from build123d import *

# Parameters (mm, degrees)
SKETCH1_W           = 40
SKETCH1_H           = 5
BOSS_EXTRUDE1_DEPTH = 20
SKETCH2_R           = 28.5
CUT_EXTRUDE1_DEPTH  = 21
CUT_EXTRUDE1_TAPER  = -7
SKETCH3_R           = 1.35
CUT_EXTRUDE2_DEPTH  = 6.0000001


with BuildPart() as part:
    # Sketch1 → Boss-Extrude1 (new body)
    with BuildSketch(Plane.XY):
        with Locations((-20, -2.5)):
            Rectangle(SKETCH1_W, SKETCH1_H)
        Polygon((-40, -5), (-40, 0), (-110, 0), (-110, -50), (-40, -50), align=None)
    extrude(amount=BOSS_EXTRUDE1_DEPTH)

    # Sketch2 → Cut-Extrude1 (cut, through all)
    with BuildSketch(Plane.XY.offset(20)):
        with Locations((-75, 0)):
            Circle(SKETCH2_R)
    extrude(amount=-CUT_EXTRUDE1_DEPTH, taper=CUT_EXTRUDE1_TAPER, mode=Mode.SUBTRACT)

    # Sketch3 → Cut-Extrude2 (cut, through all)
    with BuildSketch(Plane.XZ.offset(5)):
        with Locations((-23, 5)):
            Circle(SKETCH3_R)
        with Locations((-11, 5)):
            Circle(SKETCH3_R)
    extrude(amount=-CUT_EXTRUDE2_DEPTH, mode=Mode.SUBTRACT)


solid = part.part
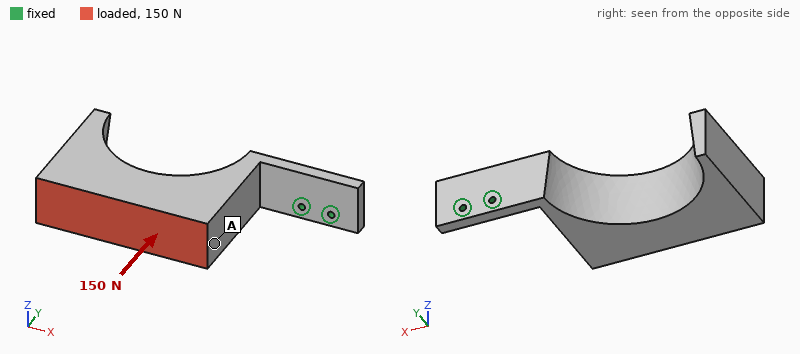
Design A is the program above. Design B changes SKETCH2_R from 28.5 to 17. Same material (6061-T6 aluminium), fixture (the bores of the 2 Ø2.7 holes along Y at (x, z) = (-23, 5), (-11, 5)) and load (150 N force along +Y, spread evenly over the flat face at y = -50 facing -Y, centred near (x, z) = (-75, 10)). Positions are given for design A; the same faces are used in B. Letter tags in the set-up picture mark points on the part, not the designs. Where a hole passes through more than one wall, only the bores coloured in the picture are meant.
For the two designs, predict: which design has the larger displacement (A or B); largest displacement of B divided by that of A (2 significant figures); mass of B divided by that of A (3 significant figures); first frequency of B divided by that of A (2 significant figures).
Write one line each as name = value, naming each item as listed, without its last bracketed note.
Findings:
which design has the larger displacement = A
largest displacement of B divided by that of A = 0.87
mass of B divided by that of A = 1.38
first frequency of B divided by that of A = 0.95
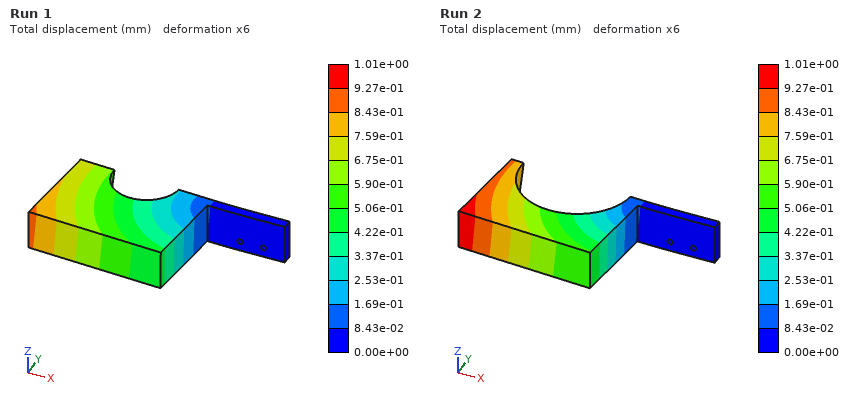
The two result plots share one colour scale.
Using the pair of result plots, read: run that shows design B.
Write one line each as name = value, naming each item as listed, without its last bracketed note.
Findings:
run that shows design B = Run 1
